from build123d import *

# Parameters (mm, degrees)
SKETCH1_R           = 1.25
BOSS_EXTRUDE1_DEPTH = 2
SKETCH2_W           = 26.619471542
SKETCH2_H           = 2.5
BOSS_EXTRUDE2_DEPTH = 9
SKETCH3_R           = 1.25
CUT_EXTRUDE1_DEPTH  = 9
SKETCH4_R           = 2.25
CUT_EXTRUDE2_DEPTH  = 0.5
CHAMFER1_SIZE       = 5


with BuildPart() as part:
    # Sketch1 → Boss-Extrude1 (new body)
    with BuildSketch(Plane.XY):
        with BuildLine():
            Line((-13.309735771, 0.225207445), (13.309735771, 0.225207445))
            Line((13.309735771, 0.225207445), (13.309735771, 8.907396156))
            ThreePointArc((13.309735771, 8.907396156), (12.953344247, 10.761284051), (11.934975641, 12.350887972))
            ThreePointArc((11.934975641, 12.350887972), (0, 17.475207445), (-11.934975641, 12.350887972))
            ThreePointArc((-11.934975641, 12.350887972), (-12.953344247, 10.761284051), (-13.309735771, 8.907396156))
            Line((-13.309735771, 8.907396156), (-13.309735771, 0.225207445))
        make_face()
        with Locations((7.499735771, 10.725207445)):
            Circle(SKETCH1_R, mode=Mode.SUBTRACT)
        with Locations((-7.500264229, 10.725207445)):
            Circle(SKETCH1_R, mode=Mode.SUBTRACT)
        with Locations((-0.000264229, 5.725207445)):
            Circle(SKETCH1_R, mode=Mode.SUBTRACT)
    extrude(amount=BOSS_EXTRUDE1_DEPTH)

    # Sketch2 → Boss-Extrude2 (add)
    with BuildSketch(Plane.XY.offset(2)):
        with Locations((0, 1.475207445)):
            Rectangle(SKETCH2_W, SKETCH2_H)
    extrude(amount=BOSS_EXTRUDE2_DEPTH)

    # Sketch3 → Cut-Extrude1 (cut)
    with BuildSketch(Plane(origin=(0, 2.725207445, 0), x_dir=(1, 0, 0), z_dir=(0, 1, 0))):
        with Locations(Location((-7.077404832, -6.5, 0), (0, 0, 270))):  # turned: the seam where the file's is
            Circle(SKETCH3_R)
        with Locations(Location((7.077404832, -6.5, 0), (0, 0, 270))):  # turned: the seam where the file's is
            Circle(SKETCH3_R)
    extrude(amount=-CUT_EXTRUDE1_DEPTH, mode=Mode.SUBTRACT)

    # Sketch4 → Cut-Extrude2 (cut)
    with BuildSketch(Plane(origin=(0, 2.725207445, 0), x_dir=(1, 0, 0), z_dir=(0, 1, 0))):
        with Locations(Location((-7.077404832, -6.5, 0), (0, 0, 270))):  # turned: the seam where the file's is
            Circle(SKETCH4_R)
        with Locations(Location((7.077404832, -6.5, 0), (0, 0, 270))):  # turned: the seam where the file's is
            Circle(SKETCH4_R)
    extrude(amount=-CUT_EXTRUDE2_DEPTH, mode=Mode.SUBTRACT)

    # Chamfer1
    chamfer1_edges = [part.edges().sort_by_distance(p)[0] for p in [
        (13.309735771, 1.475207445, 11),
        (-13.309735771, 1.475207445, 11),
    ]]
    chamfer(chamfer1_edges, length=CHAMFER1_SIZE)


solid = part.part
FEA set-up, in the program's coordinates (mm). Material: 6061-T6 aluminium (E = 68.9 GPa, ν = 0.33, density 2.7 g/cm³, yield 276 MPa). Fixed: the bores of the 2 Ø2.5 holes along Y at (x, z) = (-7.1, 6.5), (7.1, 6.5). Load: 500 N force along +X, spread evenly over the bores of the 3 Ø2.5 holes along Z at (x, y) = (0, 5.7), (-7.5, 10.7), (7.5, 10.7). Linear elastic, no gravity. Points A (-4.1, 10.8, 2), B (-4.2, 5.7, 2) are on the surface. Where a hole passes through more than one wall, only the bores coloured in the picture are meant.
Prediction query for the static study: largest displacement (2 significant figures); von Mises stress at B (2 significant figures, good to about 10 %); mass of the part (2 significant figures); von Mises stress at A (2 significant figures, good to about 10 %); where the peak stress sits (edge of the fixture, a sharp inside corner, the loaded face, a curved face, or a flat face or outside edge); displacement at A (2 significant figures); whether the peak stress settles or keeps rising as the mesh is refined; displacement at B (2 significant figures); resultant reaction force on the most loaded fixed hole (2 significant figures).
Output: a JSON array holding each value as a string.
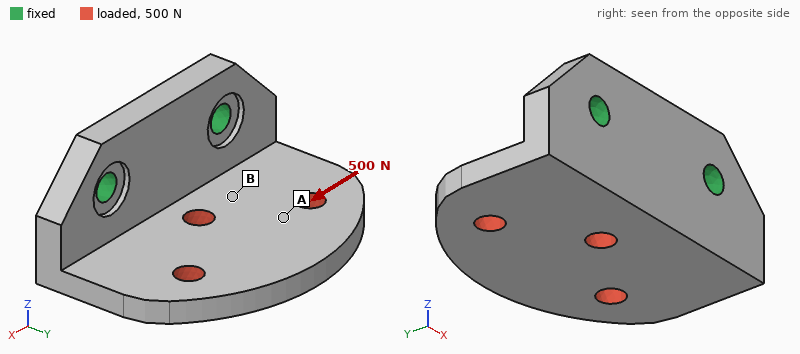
["38 µm", "42 MPa", "3.5 g", "20 MPa", "edge of the fixture", "24 µm", "keeps rising", "14 µm", "380 N"]
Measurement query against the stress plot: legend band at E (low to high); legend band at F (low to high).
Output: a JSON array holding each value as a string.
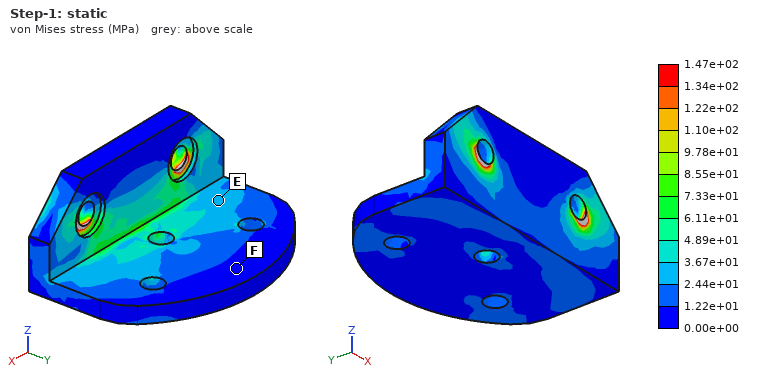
["2.44e+01 to 3.67e+01 MPa", "0.00e+00 to 1.22e+01 MPa"]
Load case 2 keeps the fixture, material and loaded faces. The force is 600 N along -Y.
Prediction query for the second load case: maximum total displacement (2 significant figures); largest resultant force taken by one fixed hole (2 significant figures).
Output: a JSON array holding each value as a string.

["95 µm", "300 N"]
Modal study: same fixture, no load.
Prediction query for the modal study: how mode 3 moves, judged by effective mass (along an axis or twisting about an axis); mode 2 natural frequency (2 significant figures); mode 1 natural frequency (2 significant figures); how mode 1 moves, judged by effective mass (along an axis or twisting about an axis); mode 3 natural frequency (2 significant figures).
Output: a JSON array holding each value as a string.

["along X", "12 kHz", "5800 Hz", "along Z", "18 kHz"]
